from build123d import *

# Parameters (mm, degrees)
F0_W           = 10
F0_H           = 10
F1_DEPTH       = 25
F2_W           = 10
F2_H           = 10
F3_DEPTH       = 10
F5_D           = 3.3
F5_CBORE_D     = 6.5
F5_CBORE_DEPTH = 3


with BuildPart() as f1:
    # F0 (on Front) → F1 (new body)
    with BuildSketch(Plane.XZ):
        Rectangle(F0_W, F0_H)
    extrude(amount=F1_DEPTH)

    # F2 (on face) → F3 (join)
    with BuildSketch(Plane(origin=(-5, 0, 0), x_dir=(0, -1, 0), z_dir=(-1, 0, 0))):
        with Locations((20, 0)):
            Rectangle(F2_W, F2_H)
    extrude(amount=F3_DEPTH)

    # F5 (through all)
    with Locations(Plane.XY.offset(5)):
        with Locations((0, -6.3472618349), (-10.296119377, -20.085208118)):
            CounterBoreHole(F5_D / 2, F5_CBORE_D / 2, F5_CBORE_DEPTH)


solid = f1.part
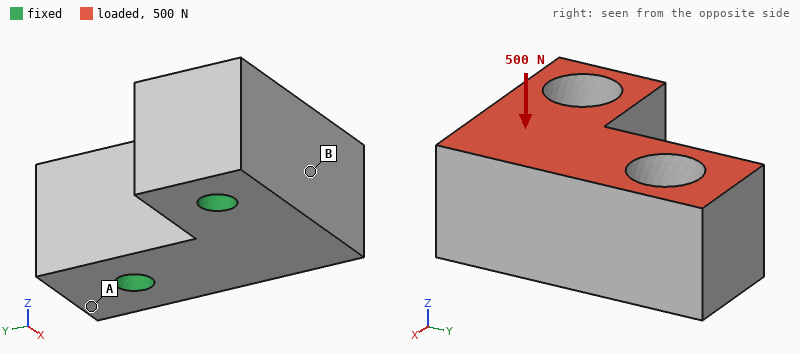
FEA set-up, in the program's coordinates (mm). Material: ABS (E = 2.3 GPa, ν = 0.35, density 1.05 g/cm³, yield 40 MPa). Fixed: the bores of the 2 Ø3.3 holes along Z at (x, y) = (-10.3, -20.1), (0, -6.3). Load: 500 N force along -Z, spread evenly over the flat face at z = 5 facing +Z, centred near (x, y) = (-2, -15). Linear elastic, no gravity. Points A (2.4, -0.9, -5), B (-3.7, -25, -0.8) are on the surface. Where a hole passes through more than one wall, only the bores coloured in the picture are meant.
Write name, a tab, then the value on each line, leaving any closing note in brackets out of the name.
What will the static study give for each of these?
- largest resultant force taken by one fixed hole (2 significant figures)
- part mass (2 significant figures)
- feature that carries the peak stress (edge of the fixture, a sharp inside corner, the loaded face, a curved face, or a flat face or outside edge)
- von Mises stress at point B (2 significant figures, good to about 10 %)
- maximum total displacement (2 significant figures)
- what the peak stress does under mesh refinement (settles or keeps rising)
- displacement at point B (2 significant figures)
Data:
largest resultant force taken by one fixed hole	260 N
part mass	3.3 g
feature that carries the peak stress	edge of the fixture
von Mises stress at point B	4.9 MPa
maximum total displacement	0.11 mm
what the peak stress does under mesh refinement	keeps rising
displacement at point B	0.047 mm
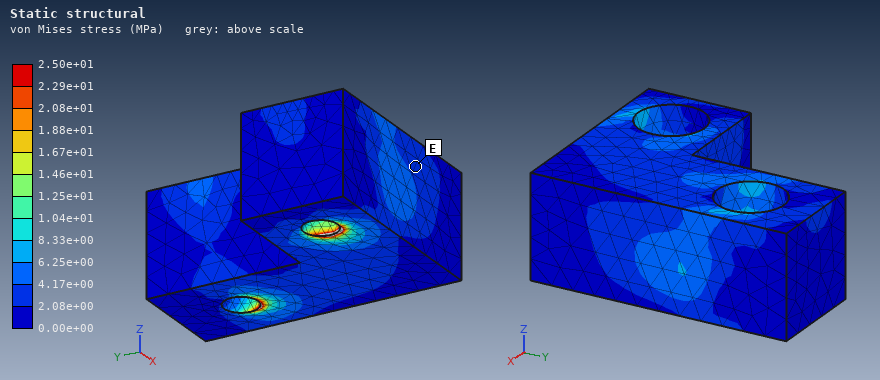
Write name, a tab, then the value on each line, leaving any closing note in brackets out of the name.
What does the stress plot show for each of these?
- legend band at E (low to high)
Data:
legend band at E	2.08e+00 to 4.17e+00 MPa
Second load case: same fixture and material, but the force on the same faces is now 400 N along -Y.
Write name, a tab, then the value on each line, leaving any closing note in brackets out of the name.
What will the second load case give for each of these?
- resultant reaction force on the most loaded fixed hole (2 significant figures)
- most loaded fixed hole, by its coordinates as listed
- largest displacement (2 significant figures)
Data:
resultant reaction force on the most loaded fixed hole	290 N
most loaded fixed hole, by its coordinates as listed	(0, -6.3)
largest displacement	83 µm
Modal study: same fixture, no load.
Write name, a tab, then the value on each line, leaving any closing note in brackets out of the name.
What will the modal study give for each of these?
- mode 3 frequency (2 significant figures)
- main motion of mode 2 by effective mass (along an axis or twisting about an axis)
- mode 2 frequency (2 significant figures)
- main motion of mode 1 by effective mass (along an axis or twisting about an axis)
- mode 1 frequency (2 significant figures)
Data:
mode 3 frequency	18 kHz
main motion of mode 2 by effective mass	along Y
mode 2 frequency	17 kHz
main motion of mode 1 by effective mass	along Z
mode 1 frequency	8200 Hz
